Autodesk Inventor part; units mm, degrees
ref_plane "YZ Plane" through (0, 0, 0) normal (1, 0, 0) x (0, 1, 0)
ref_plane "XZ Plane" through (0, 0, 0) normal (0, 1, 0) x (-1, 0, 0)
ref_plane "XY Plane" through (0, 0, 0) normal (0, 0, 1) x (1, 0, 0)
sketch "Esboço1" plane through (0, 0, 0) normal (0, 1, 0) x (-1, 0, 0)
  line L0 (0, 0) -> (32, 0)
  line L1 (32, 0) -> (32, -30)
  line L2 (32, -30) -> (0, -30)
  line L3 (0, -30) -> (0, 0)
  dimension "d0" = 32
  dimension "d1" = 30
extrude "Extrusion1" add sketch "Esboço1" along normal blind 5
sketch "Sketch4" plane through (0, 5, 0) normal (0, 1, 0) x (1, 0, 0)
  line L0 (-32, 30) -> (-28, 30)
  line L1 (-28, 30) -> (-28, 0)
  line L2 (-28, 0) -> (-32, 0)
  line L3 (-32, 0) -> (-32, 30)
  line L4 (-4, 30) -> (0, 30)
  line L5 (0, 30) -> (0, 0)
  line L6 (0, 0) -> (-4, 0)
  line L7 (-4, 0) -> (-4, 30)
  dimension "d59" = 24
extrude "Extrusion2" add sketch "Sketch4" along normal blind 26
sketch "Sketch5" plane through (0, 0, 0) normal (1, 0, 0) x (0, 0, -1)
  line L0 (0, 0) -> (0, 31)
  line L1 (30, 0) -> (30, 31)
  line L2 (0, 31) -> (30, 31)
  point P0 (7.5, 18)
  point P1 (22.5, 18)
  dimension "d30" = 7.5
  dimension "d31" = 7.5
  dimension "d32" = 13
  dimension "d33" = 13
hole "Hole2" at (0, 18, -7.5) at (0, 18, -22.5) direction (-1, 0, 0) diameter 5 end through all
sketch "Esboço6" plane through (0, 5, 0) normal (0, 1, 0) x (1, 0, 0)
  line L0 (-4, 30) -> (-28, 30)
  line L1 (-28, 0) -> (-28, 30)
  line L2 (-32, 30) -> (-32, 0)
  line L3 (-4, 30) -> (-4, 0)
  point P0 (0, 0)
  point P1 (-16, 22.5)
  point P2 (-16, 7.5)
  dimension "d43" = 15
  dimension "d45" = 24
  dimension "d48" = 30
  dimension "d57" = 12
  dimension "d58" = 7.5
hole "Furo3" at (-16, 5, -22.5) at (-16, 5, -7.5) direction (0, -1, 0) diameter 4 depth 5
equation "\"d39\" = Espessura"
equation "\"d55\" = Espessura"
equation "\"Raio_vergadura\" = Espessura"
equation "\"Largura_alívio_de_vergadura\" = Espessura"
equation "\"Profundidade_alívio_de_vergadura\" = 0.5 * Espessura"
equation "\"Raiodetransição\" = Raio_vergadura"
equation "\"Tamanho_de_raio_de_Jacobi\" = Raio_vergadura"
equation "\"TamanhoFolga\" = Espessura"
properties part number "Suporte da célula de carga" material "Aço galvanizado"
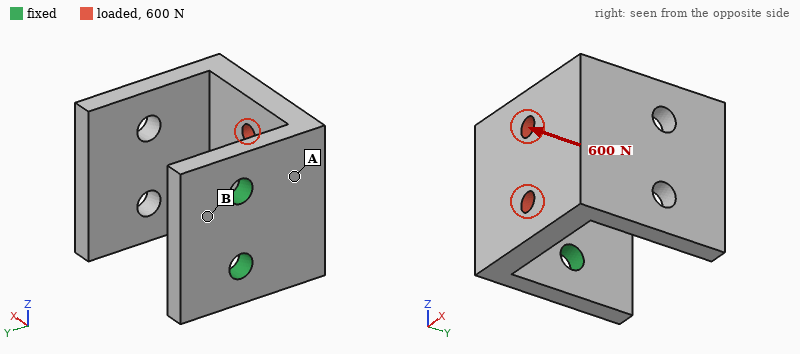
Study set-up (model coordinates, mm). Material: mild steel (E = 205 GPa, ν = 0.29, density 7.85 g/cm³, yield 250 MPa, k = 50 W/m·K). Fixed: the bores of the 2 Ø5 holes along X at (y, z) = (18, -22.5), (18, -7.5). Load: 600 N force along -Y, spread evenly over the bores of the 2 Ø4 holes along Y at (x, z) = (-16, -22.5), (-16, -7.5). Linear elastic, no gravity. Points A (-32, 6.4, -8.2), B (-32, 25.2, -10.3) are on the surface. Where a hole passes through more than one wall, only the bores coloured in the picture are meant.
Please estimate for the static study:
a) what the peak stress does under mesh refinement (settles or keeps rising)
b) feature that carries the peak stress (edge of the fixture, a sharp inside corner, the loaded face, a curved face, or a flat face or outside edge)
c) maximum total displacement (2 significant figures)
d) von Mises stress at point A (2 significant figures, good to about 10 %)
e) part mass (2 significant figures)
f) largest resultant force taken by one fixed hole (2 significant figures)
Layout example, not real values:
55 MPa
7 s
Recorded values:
keeps rising
edge of the fixture
0.15 mm
84 MPa
83 g
310 N
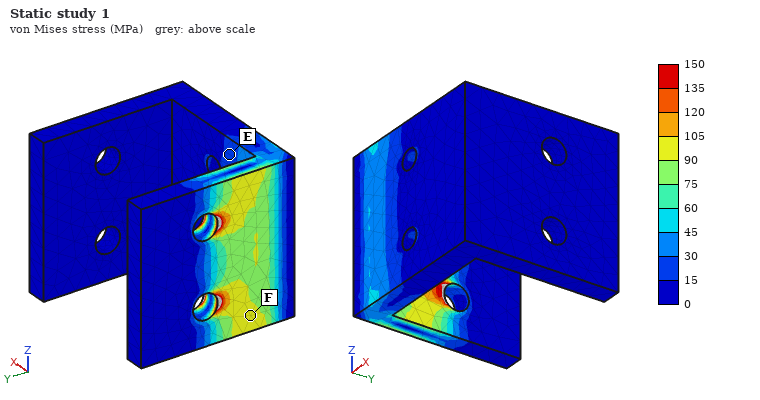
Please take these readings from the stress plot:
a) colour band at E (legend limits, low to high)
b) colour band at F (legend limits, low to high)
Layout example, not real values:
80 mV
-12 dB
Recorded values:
15 to 30 MPa
90 to 105 MPa
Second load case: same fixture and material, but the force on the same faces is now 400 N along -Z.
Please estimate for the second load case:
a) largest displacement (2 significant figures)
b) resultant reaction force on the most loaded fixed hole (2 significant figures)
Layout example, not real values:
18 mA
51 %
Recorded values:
27 µm
460 N
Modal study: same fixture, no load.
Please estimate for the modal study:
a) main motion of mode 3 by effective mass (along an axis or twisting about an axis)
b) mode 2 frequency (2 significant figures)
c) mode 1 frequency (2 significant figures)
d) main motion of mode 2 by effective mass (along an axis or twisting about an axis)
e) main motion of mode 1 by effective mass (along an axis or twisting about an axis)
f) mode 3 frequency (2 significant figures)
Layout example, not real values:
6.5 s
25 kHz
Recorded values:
along X
2000 Hz
1200 Hz
along Z
along Y
3100 Hz
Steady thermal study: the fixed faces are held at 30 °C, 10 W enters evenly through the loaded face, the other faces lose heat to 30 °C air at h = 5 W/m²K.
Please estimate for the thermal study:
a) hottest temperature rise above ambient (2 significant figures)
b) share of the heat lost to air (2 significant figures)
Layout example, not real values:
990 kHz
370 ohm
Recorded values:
41 K
7.7 %
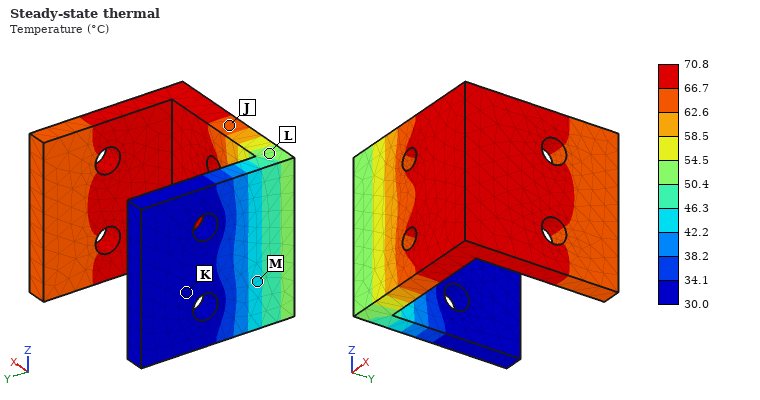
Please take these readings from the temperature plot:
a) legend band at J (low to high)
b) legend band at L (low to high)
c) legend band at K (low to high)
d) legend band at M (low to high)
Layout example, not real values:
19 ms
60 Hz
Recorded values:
62.6 to 66.7 °C
50.4 to 54.5 °C
30.0 to 34.1 °C
42.2 to 46.3 °C
